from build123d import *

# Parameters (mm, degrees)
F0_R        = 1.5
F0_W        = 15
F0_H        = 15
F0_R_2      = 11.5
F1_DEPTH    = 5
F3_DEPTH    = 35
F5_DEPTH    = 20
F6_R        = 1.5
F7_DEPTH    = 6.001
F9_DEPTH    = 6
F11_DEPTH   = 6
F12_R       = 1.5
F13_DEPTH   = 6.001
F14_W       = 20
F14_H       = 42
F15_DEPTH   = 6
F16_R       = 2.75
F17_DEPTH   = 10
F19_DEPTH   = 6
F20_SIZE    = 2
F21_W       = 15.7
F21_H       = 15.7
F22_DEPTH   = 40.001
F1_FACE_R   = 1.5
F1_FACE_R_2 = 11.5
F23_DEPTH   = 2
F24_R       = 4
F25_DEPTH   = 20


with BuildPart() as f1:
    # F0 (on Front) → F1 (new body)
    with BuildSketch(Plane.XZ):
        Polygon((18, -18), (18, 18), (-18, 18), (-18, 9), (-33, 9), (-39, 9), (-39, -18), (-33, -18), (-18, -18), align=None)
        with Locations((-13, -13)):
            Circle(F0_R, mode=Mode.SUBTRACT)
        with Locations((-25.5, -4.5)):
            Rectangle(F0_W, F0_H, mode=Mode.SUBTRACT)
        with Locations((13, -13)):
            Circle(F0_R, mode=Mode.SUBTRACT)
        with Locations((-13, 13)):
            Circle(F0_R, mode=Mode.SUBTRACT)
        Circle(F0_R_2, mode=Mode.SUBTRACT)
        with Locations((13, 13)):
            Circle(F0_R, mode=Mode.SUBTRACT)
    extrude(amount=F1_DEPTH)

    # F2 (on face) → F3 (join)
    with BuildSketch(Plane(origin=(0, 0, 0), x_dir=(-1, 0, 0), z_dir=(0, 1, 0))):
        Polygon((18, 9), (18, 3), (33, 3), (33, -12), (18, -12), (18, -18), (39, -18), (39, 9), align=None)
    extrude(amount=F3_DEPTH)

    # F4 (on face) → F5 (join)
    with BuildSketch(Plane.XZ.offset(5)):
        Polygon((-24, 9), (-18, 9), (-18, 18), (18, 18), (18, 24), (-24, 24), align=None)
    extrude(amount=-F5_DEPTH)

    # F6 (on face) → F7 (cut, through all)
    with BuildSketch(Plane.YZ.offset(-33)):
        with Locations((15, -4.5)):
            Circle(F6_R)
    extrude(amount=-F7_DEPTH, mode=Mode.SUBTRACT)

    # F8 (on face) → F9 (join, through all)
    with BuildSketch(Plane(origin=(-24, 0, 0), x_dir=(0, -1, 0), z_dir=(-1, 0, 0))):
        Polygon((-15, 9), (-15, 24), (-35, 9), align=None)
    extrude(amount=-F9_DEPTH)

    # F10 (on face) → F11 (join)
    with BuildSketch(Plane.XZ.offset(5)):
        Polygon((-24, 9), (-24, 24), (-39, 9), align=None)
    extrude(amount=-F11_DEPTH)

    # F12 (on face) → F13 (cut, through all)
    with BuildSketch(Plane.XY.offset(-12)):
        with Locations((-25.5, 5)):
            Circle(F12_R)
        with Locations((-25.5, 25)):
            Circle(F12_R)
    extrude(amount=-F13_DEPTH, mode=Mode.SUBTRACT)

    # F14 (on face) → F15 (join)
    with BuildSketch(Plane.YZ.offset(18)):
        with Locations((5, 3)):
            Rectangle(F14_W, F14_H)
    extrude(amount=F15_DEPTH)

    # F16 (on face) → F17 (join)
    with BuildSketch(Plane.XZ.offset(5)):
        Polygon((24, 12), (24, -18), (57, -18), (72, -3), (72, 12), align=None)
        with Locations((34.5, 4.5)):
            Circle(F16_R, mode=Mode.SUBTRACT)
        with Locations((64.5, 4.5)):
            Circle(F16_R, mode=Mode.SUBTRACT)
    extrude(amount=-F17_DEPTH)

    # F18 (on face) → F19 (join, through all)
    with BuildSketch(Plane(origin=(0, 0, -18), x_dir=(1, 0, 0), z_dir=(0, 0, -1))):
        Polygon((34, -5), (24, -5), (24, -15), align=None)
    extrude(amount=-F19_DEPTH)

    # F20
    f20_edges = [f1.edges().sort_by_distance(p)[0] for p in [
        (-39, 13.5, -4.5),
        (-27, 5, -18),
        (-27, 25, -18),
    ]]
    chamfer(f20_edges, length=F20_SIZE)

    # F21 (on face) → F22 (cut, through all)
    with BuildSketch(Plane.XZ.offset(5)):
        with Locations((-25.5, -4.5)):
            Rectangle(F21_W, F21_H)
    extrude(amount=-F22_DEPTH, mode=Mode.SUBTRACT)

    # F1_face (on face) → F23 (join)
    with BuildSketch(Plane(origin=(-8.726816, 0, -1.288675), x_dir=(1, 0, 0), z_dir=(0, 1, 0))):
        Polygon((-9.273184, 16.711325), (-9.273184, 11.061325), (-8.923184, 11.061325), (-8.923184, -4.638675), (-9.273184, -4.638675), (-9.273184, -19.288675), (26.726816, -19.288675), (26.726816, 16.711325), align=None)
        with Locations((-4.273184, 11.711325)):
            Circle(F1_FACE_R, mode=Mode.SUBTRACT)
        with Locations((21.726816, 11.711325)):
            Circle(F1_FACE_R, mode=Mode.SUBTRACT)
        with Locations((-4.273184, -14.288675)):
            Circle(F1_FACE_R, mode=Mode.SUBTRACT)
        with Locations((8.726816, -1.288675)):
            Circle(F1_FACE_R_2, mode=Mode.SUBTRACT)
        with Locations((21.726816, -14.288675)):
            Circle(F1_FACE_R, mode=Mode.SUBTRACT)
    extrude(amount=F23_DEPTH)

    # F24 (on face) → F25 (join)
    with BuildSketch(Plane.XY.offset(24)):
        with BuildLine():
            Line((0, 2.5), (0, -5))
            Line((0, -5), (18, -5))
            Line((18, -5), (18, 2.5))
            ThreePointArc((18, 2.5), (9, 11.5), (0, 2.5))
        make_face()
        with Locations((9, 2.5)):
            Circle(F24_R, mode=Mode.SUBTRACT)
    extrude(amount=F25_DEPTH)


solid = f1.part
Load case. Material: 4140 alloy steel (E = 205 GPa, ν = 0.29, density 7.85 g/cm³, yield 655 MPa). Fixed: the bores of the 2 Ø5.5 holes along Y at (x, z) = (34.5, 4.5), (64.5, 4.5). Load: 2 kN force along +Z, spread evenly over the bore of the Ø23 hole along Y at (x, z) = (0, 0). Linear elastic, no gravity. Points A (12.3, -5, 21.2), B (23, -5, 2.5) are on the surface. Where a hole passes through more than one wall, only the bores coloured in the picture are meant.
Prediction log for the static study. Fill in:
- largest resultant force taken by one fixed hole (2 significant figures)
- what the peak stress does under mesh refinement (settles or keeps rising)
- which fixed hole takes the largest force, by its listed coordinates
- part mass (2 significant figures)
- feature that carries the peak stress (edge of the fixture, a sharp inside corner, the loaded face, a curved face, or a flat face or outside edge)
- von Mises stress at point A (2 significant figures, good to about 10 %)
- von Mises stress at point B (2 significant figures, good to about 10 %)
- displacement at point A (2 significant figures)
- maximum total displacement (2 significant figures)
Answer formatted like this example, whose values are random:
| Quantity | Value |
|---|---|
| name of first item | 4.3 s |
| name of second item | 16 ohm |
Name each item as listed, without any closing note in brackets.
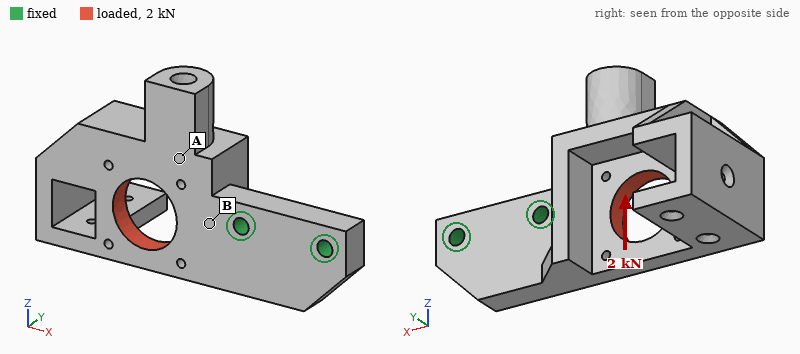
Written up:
| Quantity | Value |
|---|---|
| largest resultant force taken by one fixed hole | 4.0 kN |
| what the peak stress does under mesh refinement | keeps rising |
| which fixed hole takes the largest force, by its listed coordinates | (34.5, 4.5) |
| part mass | 380 g |
| feature that carries the peak stress | edge of the fixture |
| von Mises stress at point A | 9.7 MPa |
| von Mises stress at point B | 29 MPa |
| displacement at point A | 17 µm |
| maximum total displacement | 48 µm |
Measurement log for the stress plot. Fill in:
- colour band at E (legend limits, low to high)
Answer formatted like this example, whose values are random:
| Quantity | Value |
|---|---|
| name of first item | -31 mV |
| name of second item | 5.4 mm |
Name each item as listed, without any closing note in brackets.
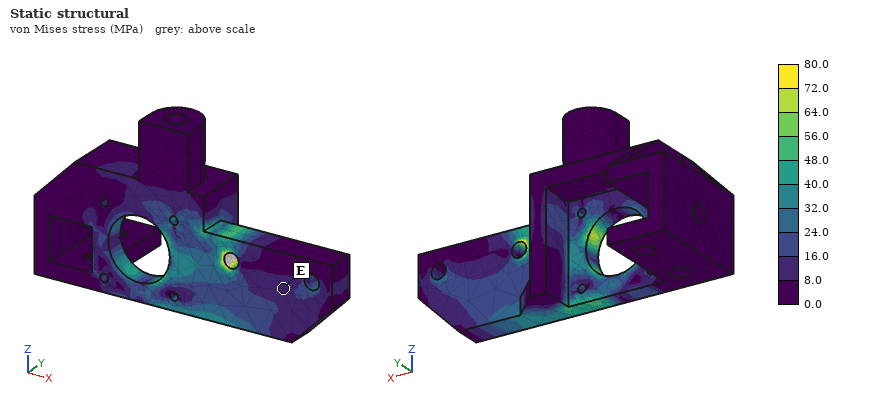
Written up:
| Quantity | Value |
|---|---|
| colour band at E | 8.0 to 16.0 MPa |
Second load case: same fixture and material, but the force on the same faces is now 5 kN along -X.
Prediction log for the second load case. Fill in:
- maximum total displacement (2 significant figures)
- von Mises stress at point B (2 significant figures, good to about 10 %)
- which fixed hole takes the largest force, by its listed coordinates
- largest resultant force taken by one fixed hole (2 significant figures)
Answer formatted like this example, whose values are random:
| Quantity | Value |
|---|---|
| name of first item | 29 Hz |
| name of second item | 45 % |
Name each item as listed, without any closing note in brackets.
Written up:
| Quantity | Value |
|---|---|
| maximum total displacement | 22 µm |
| von Mises stress at point B | 26 MPa |
| which fixed hole takes the largest force, by its listed coordinates | (34.5, 4.5) |
| largest resultant force taken by one fixed hole | 4.2 kN |
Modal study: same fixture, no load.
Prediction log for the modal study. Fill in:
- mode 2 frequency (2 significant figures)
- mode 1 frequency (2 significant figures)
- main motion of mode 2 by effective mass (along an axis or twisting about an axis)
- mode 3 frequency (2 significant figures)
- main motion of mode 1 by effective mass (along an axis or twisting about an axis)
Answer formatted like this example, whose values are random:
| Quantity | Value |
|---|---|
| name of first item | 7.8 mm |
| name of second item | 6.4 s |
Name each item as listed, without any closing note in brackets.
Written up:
| Quantity | Value |
|---|---|
| mode 2 frequency | 1400 Hz |
| mode 1 frequency | 830 Hz |
| main motion of mode 2 by effective mass | along Z |
| mode 3 frequency | 2500 Hz |
| main motion of mode 1 by effective mass | along Y |
